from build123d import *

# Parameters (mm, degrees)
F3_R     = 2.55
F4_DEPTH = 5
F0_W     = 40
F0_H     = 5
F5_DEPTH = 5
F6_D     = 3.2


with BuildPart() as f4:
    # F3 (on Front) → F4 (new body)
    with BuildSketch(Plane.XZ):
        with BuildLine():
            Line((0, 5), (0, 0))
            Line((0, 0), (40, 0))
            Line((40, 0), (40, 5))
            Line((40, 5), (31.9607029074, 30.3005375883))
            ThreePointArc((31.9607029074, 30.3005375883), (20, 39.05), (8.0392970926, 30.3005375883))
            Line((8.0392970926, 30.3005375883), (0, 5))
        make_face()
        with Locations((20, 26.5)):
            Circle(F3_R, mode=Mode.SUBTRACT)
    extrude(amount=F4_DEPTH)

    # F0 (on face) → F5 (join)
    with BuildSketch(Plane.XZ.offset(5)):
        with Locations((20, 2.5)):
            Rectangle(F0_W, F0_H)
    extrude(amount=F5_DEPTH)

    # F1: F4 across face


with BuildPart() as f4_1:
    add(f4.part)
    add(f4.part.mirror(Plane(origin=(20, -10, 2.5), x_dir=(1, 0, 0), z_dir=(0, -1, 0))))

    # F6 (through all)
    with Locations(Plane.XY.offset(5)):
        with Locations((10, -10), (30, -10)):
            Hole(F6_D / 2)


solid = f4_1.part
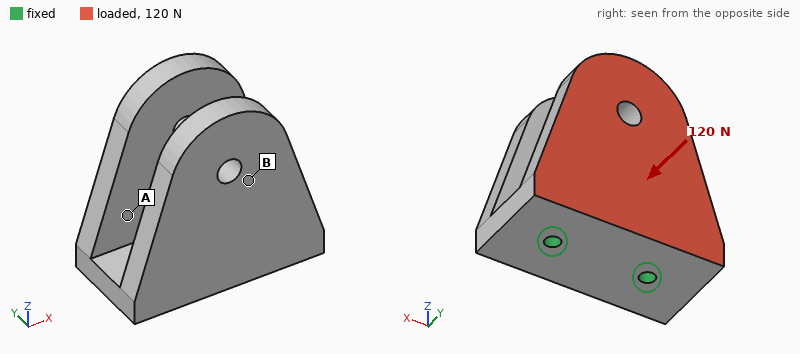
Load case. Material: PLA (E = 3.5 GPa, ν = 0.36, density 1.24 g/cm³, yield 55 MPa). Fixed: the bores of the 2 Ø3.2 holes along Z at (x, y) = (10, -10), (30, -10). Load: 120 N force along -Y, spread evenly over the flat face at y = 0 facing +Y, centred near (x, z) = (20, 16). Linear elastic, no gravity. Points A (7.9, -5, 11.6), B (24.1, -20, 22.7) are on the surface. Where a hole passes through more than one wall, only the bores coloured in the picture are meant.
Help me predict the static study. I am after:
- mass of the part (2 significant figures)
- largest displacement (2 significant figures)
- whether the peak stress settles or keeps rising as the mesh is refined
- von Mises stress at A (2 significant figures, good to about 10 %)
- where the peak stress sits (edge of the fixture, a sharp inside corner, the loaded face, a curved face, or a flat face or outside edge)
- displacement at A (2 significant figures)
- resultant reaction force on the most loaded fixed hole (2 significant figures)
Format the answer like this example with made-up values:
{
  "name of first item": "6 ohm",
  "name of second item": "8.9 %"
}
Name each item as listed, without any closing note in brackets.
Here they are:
{
  "mass of the part": "17 g",
  "largest displacement": "0.67 mm",
  "whether the peak stress settles or keeps rising as the mesh is refined": "keeps rising",
  "von Mises stress at A": "5.4 MPa",
  "where the peak stress sits": "edge of the fixture",
  "displacement at A": "0.11 mm",
  "resultant reaction force on the most loaded fixed hole": "61 N"
}
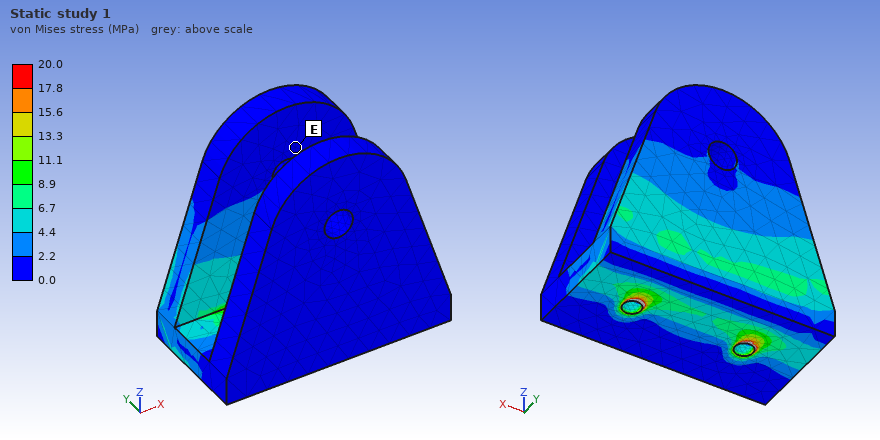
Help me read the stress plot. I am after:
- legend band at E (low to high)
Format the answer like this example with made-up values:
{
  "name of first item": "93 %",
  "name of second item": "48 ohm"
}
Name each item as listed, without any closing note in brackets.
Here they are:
{
  "legend band at E": "0.0 to 2.2 MPa"
}
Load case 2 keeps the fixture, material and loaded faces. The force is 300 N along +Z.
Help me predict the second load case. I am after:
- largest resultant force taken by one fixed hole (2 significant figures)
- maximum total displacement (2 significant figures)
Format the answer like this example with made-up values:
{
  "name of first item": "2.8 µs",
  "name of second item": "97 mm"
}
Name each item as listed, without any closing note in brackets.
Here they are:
{
  "largest resultant force taken by one fixed hole": "150 N",
  "maximum total displacement": "0.64 mm"
}
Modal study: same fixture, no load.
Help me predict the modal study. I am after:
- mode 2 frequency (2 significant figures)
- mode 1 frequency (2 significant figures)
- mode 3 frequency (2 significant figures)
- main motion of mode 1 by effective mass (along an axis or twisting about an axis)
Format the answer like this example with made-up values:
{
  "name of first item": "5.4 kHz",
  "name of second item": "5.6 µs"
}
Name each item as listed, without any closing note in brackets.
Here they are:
{
  "mode 2 frequency": "1100 Hz",
  "mode 1 frequency": "990 Hz",
  "mode 3 frequency": "2700 Hz",
  "main motion of mode 1 by effective mass": "along Y"
}
